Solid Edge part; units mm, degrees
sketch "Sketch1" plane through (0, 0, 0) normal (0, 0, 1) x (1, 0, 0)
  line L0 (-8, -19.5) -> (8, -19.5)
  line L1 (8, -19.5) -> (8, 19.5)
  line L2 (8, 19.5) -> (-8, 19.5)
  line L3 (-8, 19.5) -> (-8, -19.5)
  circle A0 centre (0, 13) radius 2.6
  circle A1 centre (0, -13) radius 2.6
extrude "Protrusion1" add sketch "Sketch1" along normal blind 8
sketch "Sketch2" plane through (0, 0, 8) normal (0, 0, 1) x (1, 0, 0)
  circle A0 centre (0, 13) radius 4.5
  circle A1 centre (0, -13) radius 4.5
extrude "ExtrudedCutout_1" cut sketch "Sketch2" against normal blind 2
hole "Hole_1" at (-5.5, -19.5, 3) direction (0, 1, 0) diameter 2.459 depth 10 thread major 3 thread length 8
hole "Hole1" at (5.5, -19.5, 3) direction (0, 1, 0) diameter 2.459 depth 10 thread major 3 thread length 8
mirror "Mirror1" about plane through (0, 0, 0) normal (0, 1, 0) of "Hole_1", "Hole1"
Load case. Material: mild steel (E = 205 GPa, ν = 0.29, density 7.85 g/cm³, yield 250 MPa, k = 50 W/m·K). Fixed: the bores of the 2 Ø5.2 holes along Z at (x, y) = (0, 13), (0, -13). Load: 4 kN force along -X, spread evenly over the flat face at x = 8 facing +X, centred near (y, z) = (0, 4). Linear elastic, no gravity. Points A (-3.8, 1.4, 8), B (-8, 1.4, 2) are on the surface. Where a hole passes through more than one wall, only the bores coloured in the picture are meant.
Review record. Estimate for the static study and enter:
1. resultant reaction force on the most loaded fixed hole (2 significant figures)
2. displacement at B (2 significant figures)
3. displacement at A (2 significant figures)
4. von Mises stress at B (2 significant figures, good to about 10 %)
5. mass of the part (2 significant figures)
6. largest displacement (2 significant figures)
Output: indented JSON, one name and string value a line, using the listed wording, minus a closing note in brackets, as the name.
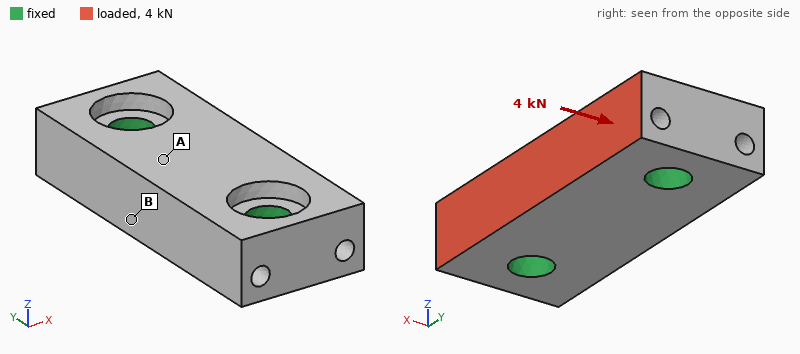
{
  "resultant reaction force on the most loaded fixed hole": "2.0 kN",
  "displacement at B": "1.2 µm",
  "displacement at A": "1.6 µm",
  "von Mises stress at B": "15 MPa",
  "mass of the part": "34 g",
  "largest displacement": "2.2 µm"
}
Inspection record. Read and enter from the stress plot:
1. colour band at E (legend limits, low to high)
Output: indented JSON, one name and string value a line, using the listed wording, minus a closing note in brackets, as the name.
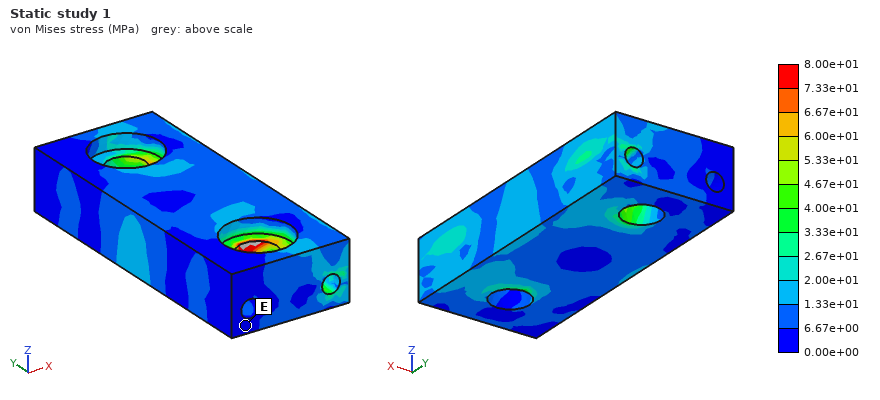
{
  "colour band at E": "0.00e+00 to 6.67e+00 MPa"
}
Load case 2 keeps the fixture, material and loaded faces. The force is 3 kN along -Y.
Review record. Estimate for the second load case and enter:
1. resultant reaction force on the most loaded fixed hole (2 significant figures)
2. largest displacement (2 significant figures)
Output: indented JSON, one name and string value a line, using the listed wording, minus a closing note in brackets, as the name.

{
  "resultant reaction force on the most loaded fixed hole": "1.7 kN",
  "largest displacement": "2.5 µm"
}
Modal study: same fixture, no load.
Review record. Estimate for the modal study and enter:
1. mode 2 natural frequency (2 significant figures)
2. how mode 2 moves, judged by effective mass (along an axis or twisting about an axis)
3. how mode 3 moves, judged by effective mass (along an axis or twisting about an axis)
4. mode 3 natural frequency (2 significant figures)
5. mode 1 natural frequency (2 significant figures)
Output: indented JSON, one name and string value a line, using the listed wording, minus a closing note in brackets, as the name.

{
  "mode 2 natural frequency": "38 kHz",
  "how mode 2 moves, judged by effective mass": "along Z",
  "how mode 3 moves, judged by effective mass": "along X",
  "mode 3 natural frequency": "47 kHz",
  "mode 1 natural frequency": "36 kHz"
}
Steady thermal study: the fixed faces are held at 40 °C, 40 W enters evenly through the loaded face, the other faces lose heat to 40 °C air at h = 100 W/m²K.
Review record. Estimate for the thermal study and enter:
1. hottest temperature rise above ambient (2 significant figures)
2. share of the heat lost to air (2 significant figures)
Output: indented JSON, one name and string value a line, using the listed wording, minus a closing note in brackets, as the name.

{
  "hottest temperature rise above ambient": "31 K",
  "share of the heat lost to air": "5.3 %"
}
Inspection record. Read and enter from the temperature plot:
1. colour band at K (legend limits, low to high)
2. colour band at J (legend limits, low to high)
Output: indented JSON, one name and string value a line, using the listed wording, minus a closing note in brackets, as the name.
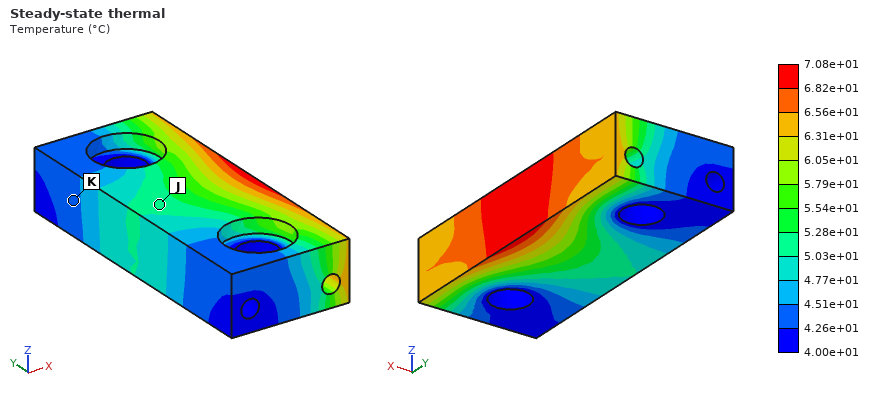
{
  "colour band at K": "4.26e+01 to 4.51e+01 °C",
  "colour band at J": "5.03e+01 to 5.28e+01 °C"
}
